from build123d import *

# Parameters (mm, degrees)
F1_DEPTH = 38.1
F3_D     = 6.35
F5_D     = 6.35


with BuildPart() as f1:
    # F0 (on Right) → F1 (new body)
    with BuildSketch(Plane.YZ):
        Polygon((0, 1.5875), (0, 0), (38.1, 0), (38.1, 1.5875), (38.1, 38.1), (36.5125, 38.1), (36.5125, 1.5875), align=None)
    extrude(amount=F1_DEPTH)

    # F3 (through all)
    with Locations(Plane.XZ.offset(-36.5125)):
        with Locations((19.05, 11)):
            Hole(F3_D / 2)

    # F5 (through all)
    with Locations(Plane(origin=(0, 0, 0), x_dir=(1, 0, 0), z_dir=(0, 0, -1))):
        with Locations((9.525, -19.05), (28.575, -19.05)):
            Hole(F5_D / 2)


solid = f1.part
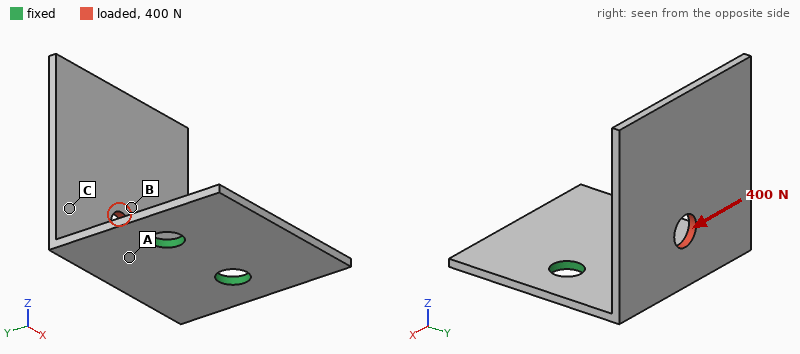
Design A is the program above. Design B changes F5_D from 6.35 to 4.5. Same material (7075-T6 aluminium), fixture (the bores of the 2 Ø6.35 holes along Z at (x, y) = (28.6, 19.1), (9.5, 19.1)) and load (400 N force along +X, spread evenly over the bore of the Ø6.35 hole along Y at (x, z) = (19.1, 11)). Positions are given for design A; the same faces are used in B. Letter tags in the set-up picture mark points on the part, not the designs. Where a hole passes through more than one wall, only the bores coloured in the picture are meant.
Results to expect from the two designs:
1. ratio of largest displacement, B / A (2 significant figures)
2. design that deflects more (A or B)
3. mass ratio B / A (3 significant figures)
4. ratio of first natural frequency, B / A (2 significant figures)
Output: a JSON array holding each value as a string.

["1.1", "B", "1.01", "0.97"]
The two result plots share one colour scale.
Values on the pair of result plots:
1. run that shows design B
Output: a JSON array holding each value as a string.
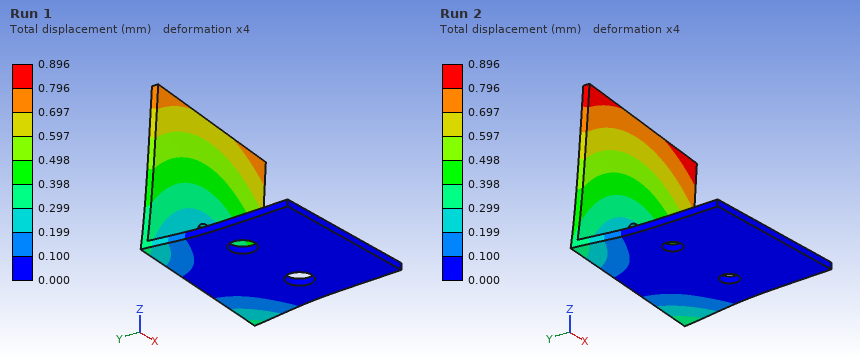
["Run 2"]
